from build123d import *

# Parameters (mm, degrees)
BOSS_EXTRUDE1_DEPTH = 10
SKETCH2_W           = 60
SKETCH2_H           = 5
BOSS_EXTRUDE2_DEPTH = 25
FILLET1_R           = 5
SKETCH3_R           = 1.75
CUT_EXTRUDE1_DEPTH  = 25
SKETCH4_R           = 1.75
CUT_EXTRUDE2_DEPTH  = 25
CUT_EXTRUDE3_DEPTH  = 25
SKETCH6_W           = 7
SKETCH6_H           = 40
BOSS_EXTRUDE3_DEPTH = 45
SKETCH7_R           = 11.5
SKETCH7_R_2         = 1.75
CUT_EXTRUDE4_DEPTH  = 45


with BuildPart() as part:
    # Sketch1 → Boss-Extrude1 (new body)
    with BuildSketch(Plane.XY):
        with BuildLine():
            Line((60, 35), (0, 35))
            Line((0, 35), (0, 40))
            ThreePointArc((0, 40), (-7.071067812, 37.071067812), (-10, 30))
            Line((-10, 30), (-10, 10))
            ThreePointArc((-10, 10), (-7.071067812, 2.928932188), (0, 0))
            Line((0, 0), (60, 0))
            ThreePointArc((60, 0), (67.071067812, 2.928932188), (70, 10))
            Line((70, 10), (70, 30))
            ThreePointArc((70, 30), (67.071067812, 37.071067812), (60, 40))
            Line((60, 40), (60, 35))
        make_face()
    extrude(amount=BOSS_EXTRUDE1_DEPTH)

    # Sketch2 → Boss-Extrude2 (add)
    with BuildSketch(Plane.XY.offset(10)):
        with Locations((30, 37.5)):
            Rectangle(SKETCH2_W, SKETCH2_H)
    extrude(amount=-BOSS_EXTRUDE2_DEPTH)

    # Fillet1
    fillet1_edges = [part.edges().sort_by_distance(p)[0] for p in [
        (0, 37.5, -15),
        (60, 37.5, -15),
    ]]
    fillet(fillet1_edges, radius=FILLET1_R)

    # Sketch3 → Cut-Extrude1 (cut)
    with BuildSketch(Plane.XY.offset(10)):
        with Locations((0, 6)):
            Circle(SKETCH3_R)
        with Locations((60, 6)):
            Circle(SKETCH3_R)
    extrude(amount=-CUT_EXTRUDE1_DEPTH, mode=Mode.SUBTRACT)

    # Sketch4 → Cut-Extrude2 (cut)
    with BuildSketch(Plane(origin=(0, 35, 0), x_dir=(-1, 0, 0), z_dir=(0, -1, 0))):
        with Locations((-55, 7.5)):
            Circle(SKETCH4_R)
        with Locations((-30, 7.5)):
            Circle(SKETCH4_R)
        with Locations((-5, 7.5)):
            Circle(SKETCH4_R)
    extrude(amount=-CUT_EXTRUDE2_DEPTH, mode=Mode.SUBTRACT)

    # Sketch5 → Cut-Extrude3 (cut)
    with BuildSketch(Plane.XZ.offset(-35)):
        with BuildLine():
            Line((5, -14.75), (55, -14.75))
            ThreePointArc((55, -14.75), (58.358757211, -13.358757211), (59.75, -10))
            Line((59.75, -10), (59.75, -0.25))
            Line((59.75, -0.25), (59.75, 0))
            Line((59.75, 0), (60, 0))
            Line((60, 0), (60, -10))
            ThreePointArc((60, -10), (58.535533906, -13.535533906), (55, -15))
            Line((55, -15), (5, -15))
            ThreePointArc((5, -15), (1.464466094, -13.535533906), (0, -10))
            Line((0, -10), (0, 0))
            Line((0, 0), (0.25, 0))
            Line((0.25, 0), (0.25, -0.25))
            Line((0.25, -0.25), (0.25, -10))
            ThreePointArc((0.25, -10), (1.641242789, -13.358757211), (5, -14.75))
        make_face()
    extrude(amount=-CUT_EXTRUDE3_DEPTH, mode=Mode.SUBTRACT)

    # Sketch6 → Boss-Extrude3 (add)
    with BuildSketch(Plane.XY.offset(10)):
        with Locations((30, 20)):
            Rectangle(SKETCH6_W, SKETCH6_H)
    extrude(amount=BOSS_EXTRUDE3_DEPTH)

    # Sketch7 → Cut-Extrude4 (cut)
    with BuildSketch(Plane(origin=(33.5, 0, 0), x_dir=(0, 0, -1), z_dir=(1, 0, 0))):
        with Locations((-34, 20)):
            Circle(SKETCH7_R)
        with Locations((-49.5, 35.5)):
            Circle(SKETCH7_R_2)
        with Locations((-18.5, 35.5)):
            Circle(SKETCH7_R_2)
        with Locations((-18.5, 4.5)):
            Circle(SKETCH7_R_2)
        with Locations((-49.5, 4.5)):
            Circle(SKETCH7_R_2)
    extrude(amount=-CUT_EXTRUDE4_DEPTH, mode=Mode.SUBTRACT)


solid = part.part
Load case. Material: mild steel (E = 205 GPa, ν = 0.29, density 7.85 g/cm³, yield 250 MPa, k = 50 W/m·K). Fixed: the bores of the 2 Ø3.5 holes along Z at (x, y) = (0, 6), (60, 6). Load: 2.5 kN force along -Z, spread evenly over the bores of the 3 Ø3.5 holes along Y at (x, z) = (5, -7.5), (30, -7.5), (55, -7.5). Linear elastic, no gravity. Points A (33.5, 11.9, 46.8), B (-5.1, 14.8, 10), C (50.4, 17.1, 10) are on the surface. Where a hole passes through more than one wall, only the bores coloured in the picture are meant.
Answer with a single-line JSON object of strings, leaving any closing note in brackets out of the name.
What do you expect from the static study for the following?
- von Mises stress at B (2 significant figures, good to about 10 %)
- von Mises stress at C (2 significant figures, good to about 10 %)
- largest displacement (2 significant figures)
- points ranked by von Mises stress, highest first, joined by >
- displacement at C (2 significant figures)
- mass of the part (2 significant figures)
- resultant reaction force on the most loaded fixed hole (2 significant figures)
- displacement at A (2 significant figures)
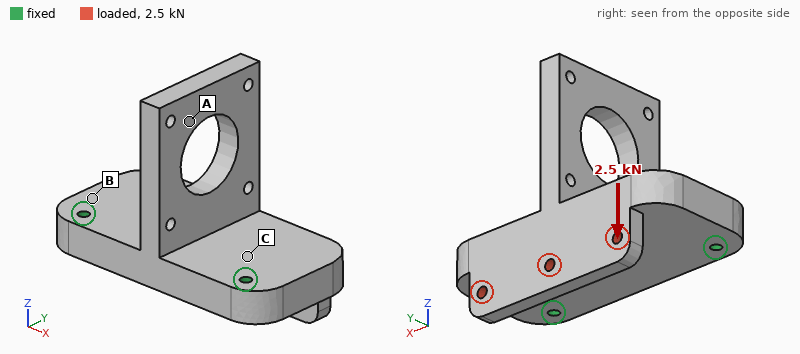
{"von Mises stress at B": "62 MPa", "von Mises stress at C": "34 MPa", "largest displacement": "82 µm", "points ranked by von Mises stress, highest first, joined by >": "B > C > A", "displacement at C": "14 µm", "mass of the part": "350 g", "resultant reaction force on the most loaded fixed hole": "1.3 kN", "displacement at A": "57 µm"}
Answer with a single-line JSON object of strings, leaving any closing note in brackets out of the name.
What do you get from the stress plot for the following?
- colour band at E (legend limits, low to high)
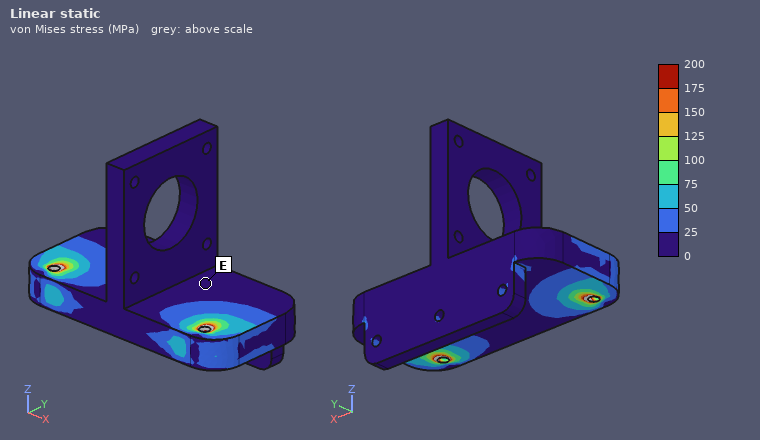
{"colour band at E": "0 to 25 MPa"}
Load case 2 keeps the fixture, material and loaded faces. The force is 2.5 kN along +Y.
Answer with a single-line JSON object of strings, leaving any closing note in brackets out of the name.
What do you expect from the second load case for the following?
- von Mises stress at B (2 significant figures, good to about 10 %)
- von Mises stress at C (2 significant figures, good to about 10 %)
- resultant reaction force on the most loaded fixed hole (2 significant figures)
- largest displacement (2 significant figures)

{"von Mises stress at B": "26 MPa", "von Mises stress at C": "16 MPa", "resultant reaction force on the most loaded fixed hole": "1.3 kN", "largest displacement": "43 µm"}
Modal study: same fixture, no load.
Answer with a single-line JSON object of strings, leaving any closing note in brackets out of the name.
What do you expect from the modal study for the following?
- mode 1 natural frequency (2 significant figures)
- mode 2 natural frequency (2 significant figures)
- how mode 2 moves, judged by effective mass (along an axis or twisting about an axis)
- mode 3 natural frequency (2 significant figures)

{"mode 1 natural frequency": "2300 Hz", "mode 2 natural frequency": "2500 Hz", "how mode 2 moves, judged by effective mass": "along Z", "mode 3 natural frequency": "5500 Hz"}
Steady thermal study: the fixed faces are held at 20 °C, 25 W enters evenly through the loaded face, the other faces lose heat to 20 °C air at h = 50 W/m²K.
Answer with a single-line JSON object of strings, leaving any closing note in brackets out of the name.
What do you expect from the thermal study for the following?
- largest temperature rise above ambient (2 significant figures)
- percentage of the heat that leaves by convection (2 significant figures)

{"largest temperature rise above ambient": "43 K", "percentage of the heat that leaves by convection": "38 %"}
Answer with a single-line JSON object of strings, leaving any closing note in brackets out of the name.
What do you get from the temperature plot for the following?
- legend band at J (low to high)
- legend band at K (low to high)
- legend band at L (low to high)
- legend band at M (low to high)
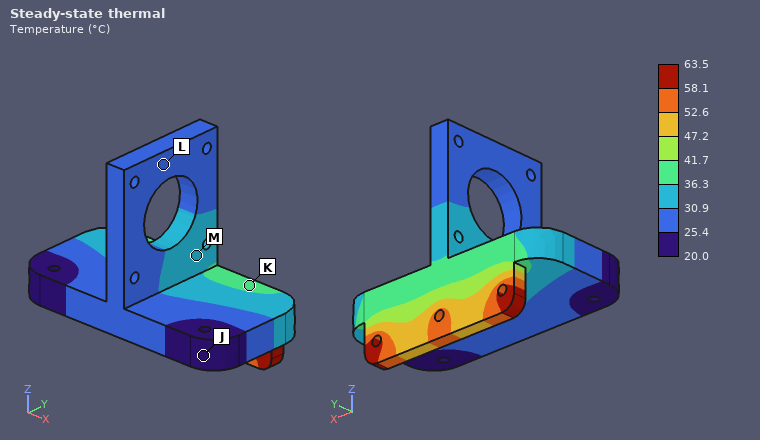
{"legend band at J": "20.0 to 25.4 °C", "legend band at K": "36.3 to 41.7 °C", "legend band at L": "25.4 to 30.9 °C", "legend band at M": "30.9 to 36.3 °C"}
